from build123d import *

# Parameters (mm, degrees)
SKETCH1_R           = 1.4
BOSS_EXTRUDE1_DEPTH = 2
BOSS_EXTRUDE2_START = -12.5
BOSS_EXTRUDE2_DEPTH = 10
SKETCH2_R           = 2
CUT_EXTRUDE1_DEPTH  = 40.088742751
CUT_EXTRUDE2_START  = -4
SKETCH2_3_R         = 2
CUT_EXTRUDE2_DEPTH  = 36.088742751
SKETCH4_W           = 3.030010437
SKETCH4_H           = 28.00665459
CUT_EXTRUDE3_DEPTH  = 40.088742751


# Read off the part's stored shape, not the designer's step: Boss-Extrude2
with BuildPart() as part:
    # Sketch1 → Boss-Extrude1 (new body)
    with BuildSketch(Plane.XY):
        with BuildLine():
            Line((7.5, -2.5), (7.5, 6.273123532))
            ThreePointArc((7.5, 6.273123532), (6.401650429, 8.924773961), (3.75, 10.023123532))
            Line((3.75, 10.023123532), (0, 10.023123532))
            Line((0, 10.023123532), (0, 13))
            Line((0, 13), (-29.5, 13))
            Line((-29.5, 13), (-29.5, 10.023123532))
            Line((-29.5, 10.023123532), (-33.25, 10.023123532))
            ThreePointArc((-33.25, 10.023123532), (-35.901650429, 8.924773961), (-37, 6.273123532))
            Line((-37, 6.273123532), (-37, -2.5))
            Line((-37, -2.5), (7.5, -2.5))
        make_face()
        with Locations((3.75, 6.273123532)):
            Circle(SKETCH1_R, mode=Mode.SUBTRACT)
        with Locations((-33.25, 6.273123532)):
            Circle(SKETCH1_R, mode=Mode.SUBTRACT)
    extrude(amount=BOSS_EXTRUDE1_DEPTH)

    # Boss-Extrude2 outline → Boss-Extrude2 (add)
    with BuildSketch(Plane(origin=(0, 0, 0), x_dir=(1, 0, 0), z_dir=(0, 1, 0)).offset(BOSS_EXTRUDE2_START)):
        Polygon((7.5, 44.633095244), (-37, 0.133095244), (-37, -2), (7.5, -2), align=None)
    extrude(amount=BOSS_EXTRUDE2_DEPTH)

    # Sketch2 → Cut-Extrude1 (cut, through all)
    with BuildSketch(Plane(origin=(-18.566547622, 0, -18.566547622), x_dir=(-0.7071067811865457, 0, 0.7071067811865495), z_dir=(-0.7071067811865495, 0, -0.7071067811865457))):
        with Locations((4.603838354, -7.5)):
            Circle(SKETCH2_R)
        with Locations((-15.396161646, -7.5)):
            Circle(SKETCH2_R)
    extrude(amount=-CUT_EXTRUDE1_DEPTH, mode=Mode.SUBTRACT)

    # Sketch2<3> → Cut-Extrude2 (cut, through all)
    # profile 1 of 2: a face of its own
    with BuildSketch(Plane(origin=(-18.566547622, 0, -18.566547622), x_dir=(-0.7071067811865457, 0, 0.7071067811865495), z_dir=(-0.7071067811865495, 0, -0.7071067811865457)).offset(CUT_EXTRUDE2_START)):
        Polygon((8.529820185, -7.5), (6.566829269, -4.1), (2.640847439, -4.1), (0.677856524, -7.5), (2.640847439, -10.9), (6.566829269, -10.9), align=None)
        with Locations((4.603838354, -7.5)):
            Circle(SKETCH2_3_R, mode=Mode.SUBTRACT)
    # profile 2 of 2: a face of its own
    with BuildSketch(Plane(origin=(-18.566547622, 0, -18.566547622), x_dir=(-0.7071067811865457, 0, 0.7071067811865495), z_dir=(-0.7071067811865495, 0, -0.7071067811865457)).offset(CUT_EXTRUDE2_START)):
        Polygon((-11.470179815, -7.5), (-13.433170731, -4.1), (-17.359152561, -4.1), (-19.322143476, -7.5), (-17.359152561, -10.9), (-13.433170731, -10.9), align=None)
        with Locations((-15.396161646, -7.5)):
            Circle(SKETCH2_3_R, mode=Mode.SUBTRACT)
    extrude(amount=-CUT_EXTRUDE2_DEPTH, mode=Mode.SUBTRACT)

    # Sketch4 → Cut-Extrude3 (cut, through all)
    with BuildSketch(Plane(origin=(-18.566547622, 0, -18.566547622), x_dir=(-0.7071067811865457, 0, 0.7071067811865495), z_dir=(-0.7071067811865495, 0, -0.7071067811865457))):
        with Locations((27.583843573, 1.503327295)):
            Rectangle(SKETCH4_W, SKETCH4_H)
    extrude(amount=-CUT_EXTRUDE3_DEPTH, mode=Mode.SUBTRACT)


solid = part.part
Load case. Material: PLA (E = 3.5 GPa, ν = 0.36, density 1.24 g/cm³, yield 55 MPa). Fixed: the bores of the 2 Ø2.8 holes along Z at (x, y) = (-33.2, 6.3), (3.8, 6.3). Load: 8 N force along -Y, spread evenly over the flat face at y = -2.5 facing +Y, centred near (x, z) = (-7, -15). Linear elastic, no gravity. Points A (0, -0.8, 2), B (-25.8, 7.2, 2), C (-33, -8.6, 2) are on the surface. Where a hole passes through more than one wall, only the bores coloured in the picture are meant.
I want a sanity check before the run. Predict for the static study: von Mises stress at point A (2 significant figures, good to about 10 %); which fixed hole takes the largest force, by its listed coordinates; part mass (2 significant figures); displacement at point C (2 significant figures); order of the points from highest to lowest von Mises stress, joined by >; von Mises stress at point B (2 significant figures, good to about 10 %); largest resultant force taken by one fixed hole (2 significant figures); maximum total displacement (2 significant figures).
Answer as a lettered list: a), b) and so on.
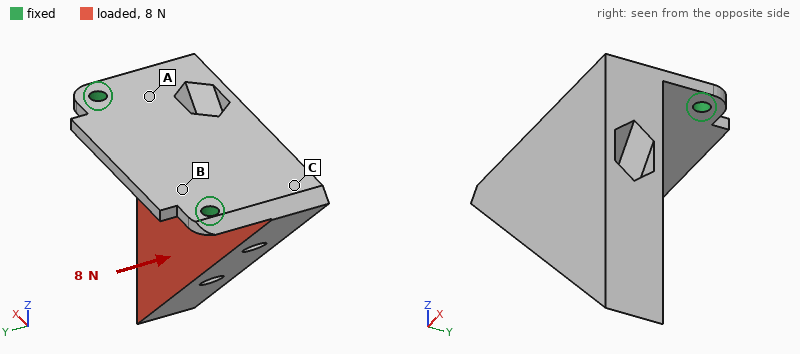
a) 4.5 MPa
b) (3.8, 6.3)
c) 13 g
d) 0.16 mm
e) A > B > C
f) 2.2 MPa
g) 5.9 N
h) 0.75 mm
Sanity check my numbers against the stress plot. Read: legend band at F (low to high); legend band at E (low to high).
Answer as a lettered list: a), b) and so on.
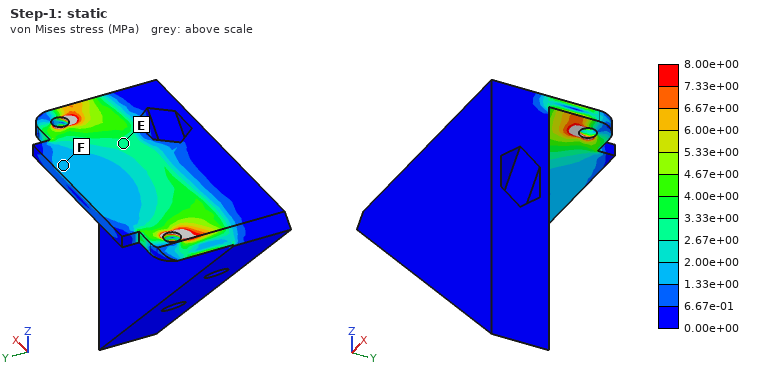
a) 1.33e+00 to 2.00e+00 MPa
b) 2.67e+00 to 3.33e+00 MPa
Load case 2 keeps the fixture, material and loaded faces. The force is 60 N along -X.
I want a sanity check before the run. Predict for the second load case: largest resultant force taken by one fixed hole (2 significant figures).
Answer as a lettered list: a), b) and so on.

a) 44 N
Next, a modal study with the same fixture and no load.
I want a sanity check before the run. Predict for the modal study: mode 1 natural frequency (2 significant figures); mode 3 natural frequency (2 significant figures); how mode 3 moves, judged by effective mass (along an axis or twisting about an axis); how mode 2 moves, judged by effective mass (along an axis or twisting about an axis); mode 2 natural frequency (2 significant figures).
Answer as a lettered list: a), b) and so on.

a) 200 Hz
b) 1300 Hz
c) along Z
d) along X
e) 880 Hz
